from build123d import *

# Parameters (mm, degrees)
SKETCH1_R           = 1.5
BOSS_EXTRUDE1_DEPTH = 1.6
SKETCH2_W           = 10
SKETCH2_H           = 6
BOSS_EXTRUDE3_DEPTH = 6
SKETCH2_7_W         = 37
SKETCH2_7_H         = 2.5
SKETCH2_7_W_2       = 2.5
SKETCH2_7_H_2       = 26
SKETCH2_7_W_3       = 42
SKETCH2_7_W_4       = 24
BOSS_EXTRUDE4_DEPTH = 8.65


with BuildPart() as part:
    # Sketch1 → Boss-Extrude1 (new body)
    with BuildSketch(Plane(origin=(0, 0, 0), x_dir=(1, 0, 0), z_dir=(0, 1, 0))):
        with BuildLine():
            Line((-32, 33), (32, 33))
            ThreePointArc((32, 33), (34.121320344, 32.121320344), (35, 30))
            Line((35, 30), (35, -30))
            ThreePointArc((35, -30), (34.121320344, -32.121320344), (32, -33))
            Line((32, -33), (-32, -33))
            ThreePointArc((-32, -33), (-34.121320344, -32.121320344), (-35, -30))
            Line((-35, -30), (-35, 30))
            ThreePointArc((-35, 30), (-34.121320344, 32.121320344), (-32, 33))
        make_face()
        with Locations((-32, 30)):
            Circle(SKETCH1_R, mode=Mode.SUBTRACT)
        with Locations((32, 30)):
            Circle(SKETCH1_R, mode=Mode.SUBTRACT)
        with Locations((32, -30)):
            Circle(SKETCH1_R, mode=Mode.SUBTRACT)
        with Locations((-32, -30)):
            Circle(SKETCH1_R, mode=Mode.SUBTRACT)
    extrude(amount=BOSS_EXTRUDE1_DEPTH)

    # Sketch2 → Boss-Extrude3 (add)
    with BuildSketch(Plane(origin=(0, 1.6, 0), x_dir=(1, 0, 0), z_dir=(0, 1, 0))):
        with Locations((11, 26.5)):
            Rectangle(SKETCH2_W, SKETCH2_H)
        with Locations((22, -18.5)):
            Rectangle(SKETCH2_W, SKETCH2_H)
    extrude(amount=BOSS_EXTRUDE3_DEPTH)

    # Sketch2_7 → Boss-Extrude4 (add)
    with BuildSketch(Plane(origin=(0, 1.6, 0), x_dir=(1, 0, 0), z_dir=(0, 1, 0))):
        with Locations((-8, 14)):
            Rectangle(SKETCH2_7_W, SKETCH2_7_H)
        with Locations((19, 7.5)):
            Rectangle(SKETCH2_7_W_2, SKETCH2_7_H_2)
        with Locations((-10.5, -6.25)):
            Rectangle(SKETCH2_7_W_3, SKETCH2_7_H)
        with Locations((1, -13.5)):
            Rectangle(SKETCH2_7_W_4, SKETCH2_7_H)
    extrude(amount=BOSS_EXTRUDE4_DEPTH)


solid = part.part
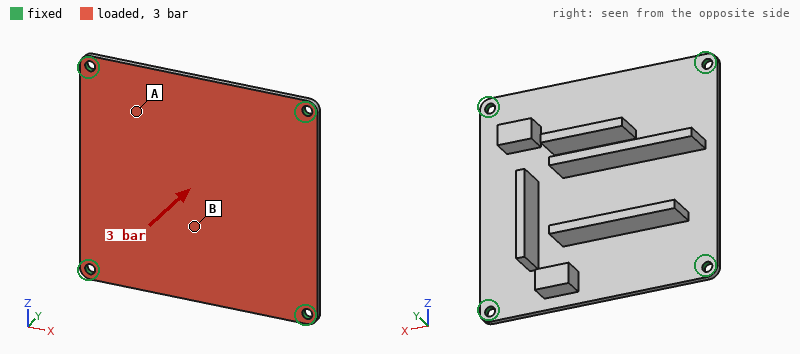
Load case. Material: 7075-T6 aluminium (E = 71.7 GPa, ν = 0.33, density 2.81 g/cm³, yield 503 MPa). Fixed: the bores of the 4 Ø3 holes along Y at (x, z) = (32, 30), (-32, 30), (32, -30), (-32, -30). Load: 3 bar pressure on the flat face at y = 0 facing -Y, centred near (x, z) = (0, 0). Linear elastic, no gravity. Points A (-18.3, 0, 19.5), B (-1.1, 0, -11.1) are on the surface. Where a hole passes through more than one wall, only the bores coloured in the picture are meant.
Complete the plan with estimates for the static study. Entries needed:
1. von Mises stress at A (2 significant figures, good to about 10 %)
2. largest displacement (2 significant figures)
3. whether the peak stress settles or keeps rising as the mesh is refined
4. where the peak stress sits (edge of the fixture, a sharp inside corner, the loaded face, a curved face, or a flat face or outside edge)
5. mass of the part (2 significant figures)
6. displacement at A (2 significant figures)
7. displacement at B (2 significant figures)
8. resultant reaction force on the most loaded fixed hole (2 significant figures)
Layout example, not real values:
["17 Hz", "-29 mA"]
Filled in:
["88 MPa", "0.80 mm", "keeps rising", "edge of the fixture", "30 g", "0.48 mm", "0.64 mm", "370 N"]
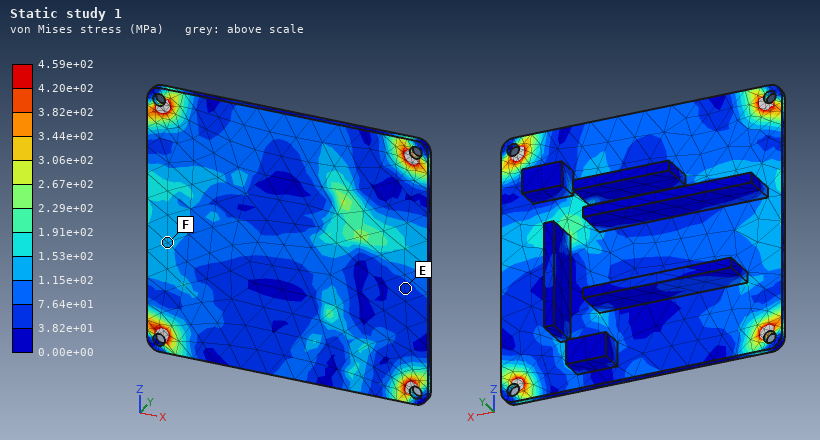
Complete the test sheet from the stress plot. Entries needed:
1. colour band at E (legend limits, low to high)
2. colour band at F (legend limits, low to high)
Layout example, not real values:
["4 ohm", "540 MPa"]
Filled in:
["3.82e+01 to 7.64e+01 MPa", "1.15e+02 to 1.53e+02 MPa"]
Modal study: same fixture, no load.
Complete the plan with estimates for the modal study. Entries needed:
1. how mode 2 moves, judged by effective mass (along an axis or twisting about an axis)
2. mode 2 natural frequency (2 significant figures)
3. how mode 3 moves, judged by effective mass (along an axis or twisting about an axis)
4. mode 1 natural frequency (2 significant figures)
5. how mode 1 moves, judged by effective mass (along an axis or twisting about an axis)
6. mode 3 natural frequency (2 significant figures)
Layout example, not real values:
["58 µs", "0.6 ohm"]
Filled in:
["twisting about Z", "2300 Hz", "twisting about X", "1300 Hz", "along Y", "2400 Hz"]
